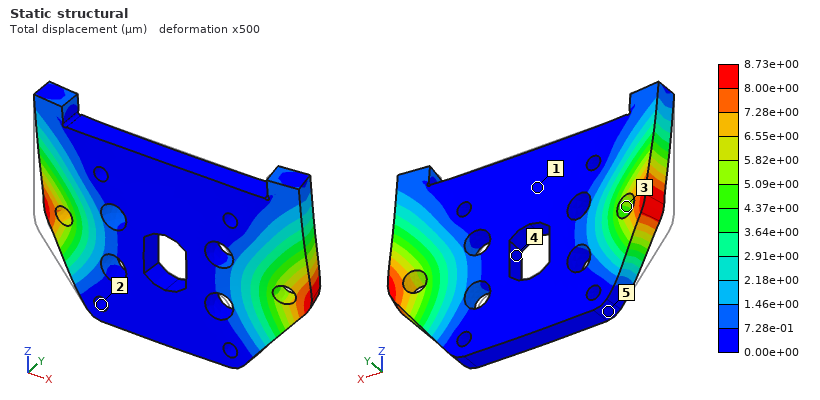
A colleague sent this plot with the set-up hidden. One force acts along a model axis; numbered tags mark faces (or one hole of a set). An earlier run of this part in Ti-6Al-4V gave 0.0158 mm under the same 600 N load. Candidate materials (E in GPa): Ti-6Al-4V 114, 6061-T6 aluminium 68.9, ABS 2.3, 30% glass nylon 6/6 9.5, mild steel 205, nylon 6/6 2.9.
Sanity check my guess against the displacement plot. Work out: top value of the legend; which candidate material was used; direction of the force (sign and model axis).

8.73e+00 µm
mild steel
+Y
